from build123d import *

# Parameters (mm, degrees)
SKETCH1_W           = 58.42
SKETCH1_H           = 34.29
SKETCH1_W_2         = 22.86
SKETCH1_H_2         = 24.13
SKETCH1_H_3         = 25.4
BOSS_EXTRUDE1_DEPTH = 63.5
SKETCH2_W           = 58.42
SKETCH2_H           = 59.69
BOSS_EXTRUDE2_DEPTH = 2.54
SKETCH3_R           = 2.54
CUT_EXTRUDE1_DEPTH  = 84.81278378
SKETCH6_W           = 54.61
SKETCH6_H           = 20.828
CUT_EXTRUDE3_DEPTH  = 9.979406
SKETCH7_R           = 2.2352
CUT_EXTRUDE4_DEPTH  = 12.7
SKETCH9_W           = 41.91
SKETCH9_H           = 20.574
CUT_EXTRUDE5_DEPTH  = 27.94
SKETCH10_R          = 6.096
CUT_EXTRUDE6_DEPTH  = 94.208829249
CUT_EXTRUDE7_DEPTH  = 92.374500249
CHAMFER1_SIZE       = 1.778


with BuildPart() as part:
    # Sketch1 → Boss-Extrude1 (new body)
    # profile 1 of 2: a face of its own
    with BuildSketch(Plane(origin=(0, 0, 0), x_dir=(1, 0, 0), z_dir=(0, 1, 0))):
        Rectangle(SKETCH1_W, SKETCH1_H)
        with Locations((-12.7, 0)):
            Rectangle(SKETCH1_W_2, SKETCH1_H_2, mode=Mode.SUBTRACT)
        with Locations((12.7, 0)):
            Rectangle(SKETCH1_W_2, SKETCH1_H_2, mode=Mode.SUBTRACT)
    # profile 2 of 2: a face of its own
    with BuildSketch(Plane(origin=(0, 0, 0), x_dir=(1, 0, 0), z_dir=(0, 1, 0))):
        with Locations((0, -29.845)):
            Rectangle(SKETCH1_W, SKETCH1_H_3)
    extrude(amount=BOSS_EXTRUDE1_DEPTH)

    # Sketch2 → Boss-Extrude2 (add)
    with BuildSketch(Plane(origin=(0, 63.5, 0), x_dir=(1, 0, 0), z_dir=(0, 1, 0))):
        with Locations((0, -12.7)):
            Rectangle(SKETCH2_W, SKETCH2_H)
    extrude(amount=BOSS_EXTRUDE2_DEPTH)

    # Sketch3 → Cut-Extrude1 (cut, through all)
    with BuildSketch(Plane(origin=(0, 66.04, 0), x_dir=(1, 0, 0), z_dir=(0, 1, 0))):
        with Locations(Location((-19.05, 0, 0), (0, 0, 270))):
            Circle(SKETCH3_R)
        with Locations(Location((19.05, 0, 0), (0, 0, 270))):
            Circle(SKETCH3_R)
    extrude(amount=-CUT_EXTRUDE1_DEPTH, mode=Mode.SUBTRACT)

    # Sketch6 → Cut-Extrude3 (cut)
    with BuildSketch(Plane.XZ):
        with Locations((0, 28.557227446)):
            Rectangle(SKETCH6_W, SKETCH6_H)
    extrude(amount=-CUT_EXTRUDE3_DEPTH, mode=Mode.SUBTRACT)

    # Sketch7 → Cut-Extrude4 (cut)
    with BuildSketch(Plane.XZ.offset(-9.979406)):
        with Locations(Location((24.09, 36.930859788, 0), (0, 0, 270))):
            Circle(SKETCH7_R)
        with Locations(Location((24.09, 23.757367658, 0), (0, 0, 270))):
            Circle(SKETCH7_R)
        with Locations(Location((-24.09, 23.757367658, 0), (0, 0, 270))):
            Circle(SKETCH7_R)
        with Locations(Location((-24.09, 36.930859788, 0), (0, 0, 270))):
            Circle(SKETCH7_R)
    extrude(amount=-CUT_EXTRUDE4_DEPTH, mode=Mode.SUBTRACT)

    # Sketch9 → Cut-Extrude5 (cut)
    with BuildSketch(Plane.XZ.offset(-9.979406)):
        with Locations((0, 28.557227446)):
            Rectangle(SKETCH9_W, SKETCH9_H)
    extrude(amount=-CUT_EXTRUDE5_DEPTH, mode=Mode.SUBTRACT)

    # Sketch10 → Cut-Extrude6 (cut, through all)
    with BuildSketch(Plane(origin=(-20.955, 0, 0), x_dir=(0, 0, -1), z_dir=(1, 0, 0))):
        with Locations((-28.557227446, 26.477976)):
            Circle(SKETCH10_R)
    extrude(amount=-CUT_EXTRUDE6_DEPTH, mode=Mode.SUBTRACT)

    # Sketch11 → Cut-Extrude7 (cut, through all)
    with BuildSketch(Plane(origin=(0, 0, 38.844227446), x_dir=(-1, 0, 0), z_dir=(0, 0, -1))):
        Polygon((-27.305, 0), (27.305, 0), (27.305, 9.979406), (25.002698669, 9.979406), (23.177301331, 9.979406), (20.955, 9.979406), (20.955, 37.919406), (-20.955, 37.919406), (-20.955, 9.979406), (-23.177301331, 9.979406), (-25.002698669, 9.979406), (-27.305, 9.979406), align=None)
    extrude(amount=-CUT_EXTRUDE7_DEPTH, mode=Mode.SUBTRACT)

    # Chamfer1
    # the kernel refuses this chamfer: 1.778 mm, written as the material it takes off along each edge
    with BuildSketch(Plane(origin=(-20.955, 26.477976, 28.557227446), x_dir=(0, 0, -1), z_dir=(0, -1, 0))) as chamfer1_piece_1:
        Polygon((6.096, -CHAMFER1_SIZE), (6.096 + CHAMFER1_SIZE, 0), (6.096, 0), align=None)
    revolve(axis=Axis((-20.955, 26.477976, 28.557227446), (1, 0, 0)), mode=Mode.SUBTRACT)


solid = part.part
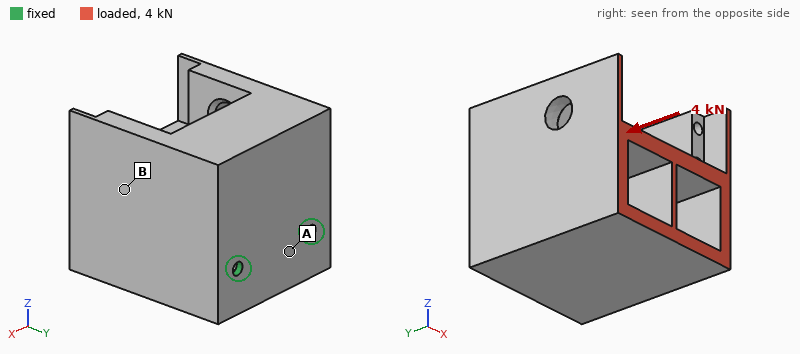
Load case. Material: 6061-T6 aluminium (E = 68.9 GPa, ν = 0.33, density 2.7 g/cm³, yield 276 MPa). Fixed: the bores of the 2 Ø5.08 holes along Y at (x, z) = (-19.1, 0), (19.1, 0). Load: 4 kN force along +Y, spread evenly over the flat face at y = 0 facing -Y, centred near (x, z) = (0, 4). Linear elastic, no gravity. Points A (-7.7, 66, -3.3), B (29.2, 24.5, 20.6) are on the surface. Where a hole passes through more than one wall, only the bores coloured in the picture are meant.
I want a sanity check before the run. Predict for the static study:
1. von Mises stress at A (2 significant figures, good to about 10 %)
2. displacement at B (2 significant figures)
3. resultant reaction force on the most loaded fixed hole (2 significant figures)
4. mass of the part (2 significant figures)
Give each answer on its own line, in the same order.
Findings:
23 MPa
0.23 mm
2.0 kN
310 g
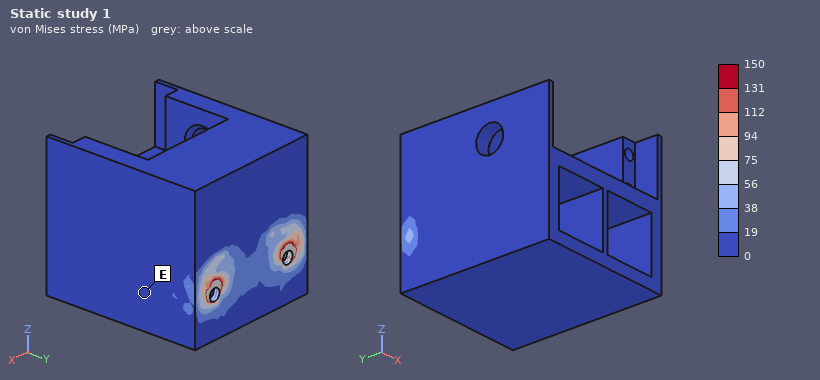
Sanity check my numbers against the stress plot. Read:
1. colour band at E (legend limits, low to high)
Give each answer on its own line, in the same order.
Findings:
0 to 19 MPa
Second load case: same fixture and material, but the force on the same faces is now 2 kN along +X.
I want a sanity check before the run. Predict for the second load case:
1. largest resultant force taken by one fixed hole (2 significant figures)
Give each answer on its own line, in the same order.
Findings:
3.1 kN
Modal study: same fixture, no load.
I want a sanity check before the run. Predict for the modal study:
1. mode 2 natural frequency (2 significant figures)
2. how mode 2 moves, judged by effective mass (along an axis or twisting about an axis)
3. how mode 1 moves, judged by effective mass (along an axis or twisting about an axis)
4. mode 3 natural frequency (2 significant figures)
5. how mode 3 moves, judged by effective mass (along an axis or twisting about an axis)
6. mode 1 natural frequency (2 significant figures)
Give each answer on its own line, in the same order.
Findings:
1800 Hz
along X
along Z
3600 Hz
along Y
410 Hz
